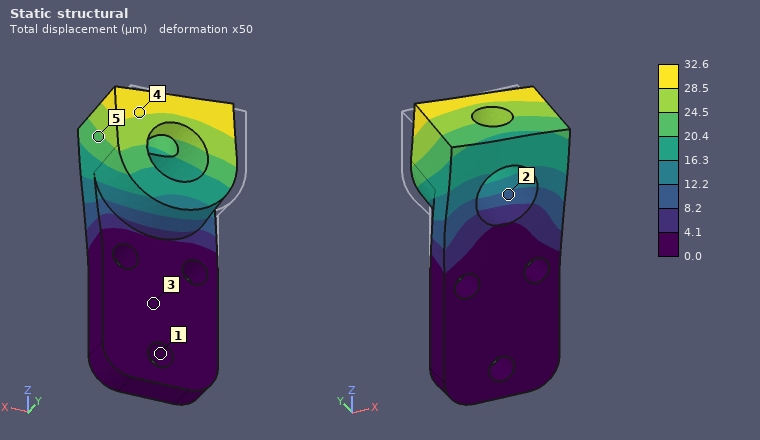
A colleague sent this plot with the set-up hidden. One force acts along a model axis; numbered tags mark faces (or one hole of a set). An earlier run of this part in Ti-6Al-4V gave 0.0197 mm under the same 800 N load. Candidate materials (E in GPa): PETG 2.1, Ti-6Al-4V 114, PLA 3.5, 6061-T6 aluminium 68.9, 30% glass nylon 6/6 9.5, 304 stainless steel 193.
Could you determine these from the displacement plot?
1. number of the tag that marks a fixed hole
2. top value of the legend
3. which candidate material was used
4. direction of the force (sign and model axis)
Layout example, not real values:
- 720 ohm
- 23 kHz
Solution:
- 1
- 32.6 µm
- 6061-T6 aluminium
- +X
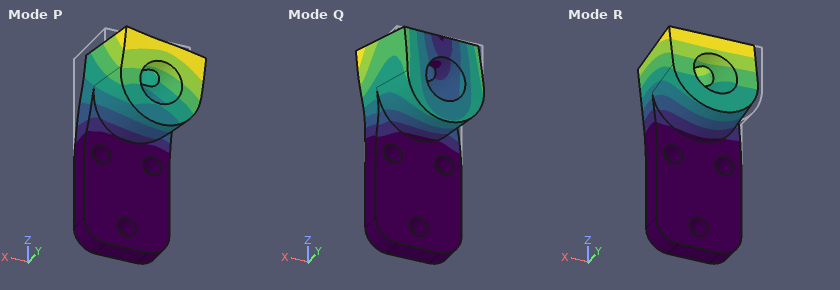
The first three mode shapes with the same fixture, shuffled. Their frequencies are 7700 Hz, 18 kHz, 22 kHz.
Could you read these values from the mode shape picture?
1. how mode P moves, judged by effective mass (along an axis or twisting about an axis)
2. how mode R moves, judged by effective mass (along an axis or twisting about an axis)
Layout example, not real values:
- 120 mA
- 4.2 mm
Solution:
- along X
- along Y
